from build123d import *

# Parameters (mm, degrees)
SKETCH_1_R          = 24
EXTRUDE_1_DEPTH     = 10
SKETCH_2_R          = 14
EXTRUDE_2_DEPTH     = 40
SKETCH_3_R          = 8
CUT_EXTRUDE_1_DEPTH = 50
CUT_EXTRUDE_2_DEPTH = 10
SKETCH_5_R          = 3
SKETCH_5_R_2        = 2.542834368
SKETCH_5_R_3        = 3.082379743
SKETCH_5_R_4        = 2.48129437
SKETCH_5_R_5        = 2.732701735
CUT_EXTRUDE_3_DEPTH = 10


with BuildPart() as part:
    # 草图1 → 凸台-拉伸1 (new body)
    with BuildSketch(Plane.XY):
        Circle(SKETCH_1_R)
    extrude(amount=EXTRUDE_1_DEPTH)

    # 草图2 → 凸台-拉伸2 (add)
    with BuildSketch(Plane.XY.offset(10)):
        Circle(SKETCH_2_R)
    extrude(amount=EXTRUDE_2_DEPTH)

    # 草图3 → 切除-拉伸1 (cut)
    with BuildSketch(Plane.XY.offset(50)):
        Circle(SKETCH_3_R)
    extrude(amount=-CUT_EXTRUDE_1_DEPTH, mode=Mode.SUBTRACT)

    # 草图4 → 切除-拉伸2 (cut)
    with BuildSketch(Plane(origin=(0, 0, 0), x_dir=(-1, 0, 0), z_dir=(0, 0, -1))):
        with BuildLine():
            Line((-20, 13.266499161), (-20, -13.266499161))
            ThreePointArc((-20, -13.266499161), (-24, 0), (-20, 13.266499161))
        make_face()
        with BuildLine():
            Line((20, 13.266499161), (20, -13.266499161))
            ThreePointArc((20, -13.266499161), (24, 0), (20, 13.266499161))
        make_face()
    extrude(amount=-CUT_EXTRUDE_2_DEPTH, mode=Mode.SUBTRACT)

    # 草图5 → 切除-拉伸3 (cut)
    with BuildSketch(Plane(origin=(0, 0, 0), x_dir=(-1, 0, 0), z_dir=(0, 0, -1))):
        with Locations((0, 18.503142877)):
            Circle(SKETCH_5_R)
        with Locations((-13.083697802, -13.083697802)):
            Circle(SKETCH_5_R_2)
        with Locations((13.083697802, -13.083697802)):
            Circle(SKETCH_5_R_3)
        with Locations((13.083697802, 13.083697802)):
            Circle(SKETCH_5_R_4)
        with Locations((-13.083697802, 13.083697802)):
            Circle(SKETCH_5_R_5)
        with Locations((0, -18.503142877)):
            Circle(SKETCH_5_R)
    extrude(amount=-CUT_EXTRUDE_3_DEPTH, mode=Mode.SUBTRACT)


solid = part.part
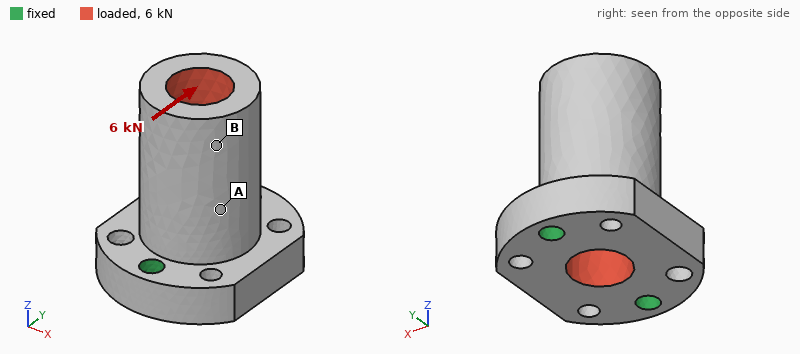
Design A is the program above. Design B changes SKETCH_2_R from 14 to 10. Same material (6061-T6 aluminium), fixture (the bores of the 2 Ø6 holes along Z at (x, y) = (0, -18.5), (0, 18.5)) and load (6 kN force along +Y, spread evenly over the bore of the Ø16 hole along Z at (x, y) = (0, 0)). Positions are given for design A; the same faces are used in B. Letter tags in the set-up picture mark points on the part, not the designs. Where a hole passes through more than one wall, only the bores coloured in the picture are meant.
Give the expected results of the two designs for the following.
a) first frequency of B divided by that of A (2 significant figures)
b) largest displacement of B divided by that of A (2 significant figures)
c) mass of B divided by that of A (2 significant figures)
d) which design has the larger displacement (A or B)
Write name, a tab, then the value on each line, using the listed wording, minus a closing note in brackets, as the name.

first frequency of B divided by that of A	1.3
largest displacement of B divided by that of A	4.4
mass of B divided by that of A	0.59
which design has the larger displacement	B
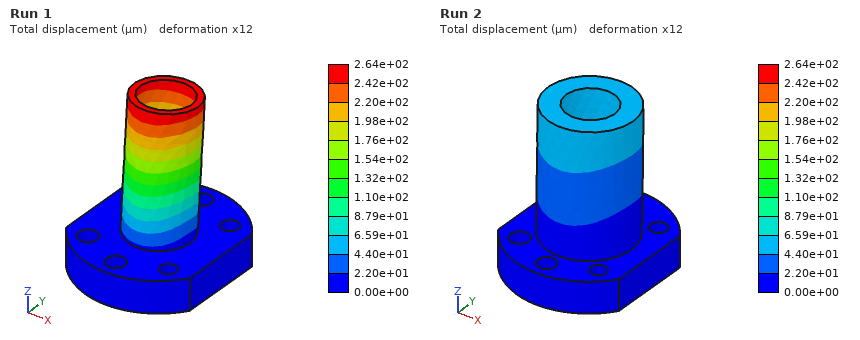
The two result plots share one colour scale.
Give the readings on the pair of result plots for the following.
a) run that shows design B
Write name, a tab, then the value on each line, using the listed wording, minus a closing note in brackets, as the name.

run that shows design B	Run 1
